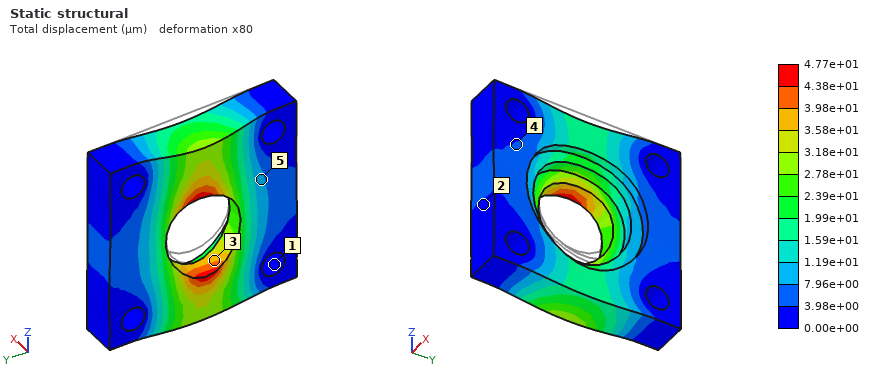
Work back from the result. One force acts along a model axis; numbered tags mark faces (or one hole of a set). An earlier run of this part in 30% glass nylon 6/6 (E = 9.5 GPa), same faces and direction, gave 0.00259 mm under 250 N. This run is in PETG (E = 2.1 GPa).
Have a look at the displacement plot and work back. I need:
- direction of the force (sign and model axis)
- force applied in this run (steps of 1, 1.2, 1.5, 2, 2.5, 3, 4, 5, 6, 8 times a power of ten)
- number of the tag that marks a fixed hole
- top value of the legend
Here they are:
-Z
1 kN
1
4.77e+01 µm
